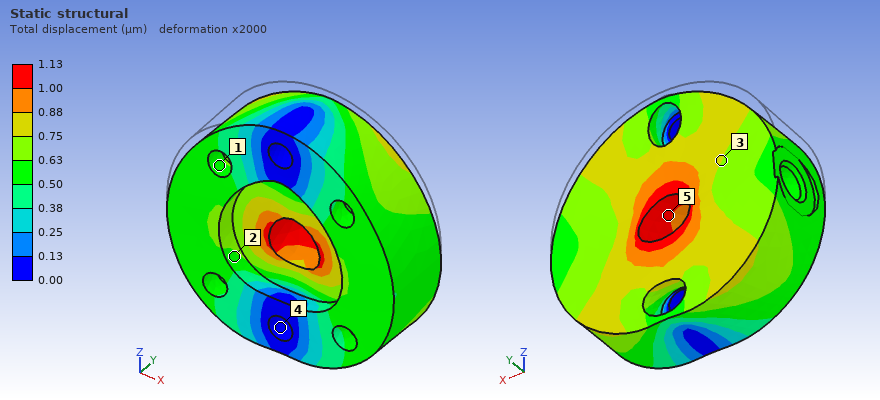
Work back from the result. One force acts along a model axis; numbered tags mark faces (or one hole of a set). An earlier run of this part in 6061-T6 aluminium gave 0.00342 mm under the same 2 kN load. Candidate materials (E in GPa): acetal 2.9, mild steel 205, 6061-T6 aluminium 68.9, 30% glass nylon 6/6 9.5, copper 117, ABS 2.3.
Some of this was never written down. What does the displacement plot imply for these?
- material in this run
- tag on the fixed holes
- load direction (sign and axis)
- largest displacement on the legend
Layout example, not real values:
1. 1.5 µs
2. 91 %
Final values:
1. mild steel
2. 4
3. -Z
4. 1.13 µm
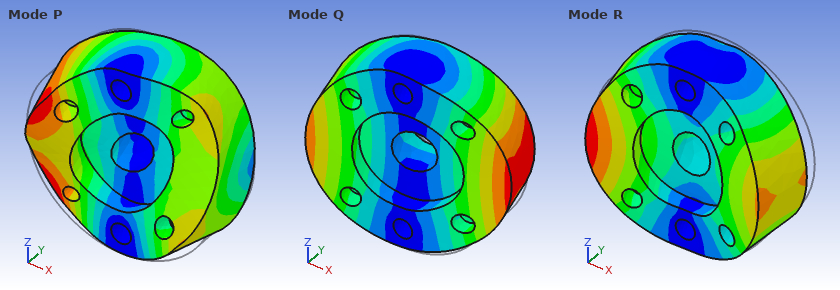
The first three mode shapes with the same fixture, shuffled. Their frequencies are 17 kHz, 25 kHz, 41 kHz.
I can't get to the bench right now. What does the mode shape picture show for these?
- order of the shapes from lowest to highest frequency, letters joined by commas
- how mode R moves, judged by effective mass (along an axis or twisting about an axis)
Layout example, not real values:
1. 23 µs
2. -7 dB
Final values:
1. Q, R, P
2. along Y
